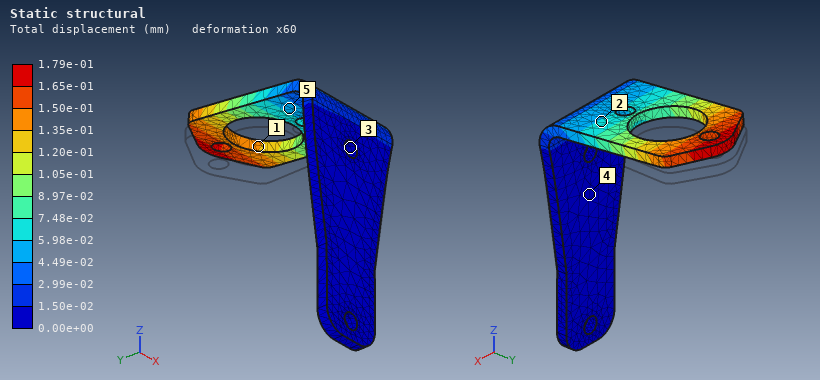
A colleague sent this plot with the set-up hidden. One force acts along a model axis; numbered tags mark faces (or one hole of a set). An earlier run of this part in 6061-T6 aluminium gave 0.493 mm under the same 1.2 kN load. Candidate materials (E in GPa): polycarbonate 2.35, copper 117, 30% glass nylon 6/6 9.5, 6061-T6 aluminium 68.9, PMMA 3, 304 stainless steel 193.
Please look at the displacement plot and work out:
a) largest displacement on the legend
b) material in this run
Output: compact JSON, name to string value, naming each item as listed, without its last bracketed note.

{"largest displacement on the legend": "1.79e-01 mm", "material in this run": "304 stainless steel"}
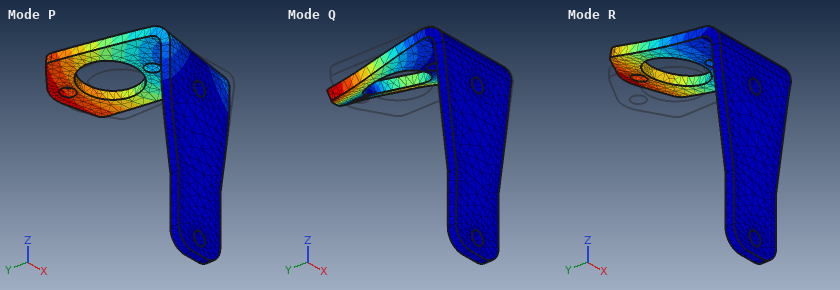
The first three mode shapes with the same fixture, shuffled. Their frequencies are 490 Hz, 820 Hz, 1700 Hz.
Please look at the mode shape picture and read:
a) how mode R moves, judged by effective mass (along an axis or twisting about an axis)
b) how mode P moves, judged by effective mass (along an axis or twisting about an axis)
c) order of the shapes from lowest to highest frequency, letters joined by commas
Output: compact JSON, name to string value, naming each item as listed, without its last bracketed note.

{"how mode R moves, judged by effective mass": "along Z", "how mode P moves, judged by effective mass": "along X", "order of the shapes from lowest to highest frequency, letters joined by commas": "R, P, Q"}
